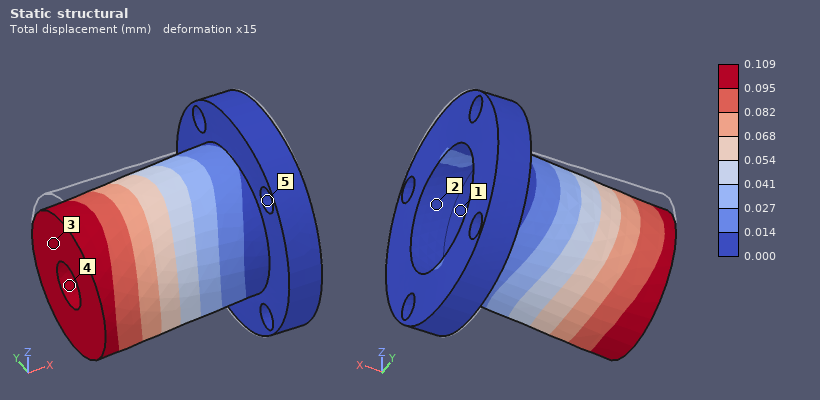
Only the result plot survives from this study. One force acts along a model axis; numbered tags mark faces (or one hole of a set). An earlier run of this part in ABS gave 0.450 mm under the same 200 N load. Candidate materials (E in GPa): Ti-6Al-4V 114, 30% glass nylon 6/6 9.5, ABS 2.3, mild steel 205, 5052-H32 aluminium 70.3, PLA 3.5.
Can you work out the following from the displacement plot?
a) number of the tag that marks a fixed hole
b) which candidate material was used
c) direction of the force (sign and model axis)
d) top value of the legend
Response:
5
30% glass nylon 6/6
-Z
0.109 mm
